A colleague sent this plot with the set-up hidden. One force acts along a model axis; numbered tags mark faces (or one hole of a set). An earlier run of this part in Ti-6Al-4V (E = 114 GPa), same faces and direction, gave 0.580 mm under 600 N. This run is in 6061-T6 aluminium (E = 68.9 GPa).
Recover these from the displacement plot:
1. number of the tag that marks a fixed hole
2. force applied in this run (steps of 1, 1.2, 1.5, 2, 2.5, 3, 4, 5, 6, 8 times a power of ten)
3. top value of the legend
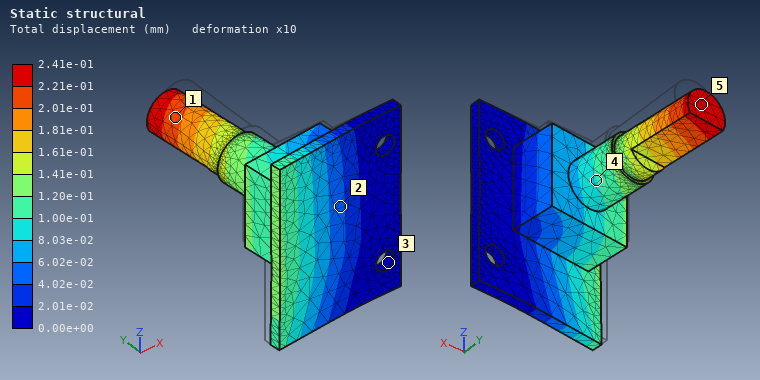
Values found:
3
150 N
2.41e-01 mm
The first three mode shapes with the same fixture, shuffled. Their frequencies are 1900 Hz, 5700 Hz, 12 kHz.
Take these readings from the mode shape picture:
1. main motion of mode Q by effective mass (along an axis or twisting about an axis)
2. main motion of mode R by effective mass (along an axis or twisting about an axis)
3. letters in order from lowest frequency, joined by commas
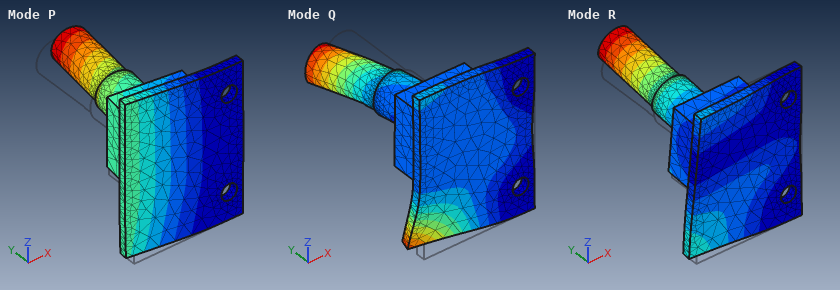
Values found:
along Y
along Z
P, R, Q
